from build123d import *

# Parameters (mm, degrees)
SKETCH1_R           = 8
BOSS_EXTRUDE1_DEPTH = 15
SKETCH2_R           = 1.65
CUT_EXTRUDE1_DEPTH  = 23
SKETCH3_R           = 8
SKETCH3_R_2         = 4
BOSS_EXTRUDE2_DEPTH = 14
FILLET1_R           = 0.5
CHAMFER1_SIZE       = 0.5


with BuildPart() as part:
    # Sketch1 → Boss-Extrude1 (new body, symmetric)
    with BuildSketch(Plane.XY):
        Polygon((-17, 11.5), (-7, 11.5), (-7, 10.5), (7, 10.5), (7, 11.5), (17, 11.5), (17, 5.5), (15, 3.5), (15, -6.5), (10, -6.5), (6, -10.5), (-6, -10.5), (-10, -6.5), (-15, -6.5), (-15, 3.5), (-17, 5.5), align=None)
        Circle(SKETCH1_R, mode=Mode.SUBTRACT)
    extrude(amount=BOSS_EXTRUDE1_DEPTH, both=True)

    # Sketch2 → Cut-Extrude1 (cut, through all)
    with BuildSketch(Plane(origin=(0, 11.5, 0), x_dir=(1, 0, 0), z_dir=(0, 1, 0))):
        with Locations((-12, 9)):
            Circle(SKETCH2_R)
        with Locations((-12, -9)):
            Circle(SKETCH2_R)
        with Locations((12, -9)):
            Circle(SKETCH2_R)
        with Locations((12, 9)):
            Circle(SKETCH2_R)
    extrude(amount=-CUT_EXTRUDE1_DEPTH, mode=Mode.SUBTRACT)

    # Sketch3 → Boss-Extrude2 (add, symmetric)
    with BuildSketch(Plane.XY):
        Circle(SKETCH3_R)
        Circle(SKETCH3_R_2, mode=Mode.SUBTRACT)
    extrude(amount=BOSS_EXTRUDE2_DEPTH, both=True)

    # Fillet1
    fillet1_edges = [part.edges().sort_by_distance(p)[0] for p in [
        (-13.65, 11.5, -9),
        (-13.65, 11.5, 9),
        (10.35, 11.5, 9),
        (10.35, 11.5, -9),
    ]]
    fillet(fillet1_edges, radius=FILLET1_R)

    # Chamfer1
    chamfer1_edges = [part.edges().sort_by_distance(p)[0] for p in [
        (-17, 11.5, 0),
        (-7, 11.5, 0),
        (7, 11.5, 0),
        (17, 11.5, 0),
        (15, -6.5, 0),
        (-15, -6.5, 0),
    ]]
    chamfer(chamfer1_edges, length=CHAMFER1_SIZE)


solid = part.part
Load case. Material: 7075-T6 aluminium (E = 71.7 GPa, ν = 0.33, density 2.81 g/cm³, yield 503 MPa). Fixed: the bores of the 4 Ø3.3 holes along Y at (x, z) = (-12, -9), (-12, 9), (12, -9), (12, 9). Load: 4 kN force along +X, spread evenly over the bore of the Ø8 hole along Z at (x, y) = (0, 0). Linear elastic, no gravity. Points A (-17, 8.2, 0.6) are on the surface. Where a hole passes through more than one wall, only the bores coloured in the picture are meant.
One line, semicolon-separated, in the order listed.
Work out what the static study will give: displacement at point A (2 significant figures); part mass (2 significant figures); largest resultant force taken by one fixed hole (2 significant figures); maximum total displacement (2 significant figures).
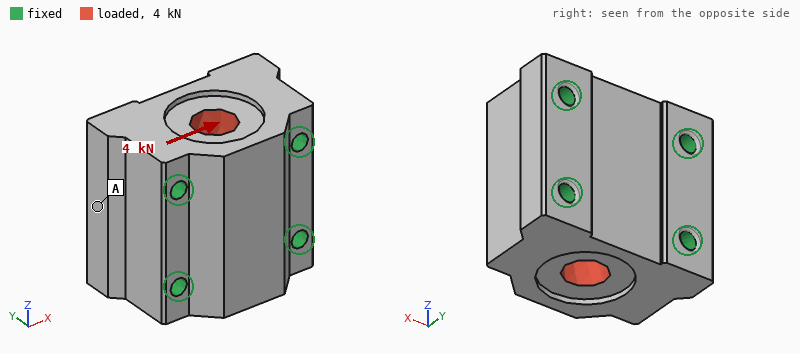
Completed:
0.37 µm; 45 g; 1.0 kN; 1.2 µm
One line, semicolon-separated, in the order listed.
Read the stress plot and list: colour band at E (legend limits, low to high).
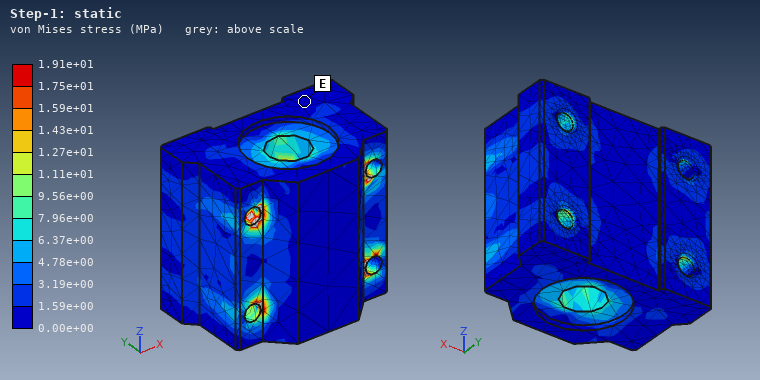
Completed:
0.00e+00 to 1.59e+00 MPa
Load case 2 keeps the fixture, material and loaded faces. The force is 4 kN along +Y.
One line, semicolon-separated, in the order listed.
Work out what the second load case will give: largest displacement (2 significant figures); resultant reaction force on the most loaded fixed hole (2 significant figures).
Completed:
2.1 µm; 1.0 kN
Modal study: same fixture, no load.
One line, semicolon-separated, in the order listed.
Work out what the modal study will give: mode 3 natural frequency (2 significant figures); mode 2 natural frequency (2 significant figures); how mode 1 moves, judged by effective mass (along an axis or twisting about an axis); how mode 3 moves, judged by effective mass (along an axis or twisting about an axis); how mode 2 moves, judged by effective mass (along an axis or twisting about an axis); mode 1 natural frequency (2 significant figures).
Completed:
62 kHz; 54 kHz; along Z; along Z; along Y; 51 kHz
